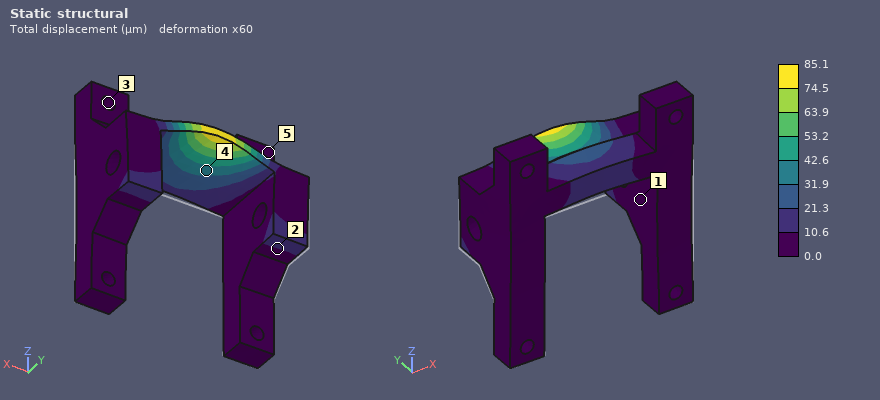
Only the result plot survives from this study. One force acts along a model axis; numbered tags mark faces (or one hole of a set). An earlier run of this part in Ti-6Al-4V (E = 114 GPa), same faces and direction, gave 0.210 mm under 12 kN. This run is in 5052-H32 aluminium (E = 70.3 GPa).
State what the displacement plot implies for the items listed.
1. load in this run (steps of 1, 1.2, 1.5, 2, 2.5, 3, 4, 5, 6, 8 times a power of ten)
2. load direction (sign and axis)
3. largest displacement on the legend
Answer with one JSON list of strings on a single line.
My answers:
["3 kN", "+Z", "85.1 µm"]
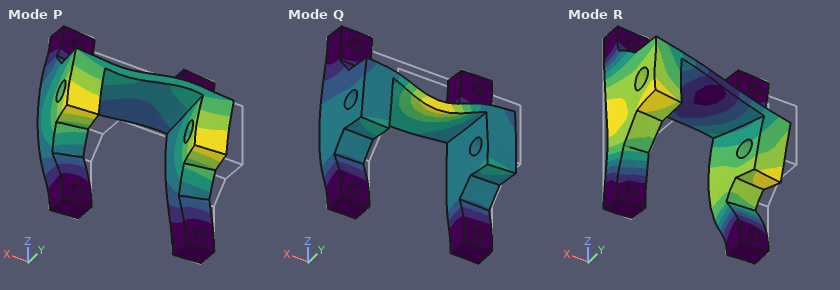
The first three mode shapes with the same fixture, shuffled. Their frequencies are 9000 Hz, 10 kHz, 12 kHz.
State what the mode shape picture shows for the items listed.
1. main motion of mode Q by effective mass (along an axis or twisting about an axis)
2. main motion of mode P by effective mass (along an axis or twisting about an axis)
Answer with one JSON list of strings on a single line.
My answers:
["along Y", "along X"]
